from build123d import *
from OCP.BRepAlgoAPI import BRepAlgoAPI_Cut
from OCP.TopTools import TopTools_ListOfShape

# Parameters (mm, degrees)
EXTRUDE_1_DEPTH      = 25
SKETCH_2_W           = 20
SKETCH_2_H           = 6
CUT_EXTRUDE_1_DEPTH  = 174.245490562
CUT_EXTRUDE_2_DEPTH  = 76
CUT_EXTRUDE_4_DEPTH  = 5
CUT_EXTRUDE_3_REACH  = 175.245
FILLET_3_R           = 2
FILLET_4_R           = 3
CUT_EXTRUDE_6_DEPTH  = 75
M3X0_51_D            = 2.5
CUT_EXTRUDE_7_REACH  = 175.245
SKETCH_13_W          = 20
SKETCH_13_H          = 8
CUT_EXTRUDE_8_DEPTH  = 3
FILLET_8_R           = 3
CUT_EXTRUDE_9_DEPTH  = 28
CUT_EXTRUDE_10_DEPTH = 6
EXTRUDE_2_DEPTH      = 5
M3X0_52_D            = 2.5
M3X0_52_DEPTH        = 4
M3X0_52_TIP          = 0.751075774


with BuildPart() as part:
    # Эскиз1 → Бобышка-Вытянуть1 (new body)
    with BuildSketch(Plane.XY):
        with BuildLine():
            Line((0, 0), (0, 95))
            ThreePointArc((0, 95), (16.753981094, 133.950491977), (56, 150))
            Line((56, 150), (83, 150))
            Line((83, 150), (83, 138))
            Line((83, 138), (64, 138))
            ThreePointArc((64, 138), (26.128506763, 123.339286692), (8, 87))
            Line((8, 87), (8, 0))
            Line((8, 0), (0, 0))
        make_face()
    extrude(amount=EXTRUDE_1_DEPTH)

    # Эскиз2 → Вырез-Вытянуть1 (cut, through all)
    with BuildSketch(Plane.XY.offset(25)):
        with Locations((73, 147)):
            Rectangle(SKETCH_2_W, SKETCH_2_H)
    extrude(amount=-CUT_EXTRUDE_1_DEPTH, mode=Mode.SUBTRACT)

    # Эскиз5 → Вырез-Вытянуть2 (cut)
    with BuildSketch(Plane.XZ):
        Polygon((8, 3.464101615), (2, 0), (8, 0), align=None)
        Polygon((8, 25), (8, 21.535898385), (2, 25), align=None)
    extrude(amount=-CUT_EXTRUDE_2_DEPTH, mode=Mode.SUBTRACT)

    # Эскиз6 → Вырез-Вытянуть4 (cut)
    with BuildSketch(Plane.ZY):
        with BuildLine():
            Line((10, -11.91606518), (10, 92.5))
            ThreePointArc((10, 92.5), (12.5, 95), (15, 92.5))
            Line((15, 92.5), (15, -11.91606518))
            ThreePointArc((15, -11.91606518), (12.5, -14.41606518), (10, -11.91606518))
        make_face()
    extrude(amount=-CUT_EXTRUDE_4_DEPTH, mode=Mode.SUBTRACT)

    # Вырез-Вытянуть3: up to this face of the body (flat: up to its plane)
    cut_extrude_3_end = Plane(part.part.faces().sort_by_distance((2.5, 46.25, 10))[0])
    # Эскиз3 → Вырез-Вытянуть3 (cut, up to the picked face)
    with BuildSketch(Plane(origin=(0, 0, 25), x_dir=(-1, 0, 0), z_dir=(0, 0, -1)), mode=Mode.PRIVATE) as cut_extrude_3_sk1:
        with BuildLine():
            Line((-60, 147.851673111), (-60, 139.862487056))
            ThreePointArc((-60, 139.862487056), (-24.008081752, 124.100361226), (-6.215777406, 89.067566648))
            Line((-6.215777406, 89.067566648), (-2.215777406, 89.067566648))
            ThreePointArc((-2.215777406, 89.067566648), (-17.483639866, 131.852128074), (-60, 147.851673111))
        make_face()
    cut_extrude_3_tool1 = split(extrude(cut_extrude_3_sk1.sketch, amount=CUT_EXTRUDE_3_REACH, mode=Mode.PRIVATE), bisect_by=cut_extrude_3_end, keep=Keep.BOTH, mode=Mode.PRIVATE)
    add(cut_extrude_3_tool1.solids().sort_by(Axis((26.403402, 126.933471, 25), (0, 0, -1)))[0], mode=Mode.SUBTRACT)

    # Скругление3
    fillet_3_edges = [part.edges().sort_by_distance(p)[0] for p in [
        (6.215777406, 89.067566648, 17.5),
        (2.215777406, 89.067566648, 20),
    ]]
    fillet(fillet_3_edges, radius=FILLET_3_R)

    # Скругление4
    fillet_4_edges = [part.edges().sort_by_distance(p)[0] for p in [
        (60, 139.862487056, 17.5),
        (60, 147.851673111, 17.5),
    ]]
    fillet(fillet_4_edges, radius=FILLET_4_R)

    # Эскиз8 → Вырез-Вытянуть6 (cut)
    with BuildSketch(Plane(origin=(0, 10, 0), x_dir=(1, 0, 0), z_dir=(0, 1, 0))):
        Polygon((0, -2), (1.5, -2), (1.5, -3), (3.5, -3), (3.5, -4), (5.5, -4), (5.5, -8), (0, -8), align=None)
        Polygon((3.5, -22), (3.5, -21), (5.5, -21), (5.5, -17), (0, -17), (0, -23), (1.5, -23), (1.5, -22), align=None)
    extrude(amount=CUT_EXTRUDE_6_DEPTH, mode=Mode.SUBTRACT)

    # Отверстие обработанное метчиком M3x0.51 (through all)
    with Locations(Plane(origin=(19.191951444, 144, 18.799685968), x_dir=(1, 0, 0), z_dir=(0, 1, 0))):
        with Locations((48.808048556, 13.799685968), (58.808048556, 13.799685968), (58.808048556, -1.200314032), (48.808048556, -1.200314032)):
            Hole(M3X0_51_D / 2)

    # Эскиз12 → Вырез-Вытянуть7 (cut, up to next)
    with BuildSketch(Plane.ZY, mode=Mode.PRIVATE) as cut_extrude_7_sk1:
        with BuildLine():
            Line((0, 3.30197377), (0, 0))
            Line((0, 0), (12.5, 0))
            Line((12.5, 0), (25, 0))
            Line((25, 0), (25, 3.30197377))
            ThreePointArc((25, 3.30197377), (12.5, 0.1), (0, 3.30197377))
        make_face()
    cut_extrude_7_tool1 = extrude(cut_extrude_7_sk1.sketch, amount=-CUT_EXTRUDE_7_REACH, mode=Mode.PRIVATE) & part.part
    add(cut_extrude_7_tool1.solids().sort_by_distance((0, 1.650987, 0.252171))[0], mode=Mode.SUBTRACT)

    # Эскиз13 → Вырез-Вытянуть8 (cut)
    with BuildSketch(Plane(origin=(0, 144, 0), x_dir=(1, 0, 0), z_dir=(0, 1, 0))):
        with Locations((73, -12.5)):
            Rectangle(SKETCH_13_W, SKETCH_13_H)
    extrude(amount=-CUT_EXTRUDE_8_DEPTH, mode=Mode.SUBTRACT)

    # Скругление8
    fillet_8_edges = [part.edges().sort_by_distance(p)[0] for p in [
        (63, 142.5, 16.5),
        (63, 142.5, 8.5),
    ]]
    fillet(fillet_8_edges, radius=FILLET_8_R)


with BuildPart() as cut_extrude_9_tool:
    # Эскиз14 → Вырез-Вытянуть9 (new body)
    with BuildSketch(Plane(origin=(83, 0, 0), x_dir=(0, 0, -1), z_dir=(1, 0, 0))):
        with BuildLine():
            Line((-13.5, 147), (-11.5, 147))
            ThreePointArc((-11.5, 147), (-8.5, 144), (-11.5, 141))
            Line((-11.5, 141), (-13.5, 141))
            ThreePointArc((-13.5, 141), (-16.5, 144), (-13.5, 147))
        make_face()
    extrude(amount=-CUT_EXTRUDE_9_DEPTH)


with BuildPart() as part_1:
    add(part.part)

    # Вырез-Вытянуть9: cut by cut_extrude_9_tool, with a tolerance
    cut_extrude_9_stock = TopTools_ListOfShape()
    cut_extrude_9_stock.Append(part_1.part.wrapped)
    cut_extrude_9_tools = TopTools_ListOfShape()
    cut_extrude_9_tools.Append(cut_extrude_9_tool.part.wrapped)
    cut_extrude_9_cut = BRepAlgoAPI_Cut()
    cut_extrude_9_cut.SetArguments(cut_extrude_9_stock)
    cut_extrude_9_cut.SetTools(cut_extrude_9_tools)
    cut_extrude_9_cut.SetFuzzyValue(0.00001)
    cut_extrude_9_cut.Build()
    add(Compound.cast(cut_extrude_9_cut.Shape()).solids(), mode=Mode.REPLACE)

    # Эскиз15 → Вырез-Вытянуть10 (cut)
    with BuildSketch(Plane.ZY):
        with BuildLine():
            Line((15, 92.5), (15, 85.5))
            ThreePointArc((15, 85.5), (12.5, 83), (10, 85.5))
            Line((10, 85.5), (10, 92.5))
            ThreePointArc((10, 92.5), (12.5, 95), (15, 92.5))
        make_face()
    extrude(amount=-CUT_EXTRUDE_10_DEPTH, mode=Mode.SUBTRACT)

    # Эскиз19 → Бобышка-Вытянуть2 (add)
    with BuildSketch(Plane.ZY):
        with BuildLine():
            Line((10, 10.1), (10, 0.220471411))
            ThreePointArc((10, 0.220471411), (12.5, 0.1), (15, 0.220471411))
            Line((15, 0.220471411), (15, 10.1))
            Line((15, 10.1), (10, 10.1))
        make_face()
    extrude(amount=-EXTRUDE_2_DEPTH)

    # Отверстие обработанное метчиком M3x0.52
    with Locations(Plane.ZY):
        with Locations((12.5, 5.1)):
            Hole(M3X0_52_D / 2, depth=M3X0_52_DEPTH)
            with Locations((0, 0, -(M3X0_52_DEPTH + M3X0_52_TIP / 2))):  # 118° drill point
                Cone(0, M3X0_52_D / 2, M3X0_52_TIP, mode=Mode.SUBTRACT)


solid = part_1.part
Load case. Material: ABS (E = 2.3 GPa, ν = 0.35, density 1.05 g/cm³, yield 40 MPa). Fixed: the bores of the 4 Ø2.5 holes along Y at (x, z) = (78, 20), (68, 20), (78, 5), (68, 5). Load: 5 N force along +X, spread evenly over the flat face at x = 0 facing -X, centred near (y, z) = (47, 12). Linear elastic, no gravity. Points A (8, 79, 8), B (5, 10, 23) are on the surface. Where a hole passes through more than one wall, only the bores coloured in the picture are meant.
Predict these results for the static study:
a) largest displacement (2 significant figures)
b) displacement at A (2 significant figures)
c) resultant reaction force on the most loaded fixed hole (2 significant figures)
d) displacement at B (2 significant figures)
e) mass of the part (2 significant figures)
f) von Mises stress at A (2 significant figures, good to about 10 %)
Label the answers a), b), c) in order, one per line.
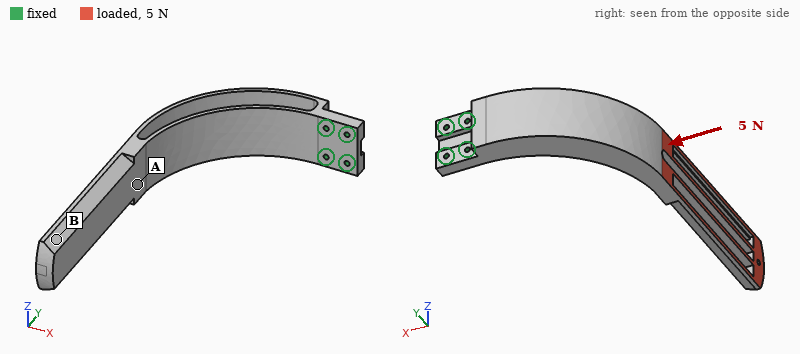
a) 1.9 mm
b) 0.72 mm
c) 8.9 N
d) 1.8 mm
e) 31 g
f) 1.0 MPa
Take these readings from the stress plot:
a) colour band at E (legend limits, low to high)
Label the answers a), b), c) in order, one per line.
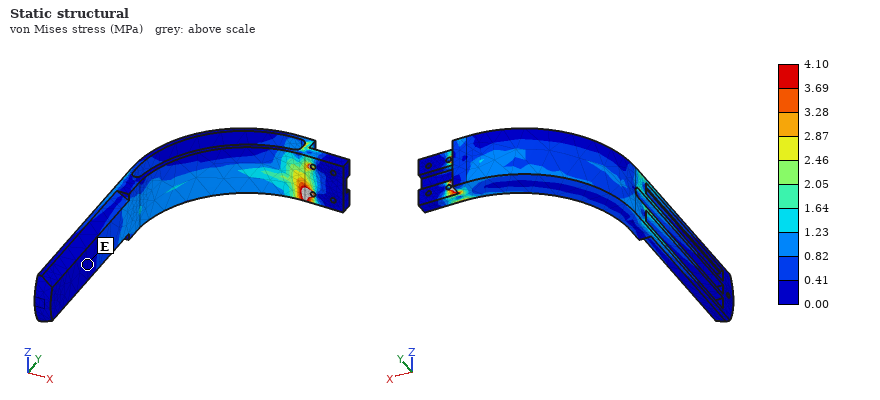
a) 0.00 to 0.41 MPa
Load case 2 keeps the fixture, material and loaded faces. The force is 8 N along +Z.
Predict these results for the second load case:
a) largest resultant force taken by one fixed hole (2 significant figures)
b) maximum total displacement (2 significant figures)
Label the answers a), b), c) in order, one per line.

a) 48 N
b) 2.0 mm
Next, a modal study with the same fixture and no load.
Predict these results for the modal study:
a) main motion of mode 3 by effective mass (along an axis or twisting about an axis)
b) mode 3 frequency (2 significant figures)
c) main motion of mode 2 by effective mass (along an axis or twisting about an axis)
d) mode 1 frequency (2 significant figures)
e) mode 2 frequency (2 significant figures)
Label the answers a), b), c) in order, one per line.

a) along Y
b) 260 Hz
c) along Z
d) 83 Hz
e) 110 Hz
